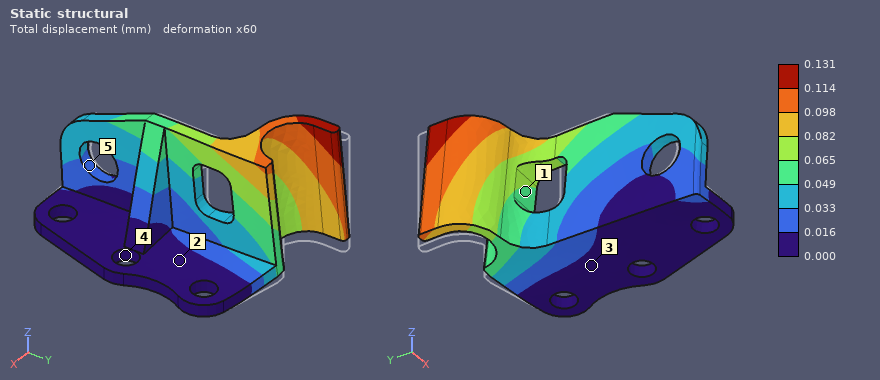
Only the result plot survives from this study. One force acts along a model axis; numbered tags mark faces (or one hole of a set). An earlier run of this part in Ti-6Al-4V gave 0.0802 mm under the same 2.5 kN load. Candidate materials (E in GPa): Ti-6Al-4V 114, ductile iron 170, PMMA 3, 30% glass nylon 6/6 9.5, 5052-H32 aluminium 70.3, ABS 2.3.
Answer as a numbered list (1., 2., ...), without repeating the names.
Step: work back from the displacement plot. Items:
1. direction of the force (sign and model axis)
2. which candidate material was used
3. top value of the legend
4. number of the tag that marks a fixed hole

1. -Y
2. 5052-H32 aluminium
3. 0.131 mm
4. 4
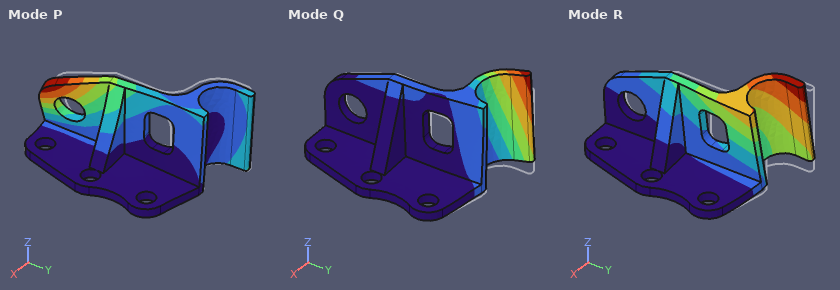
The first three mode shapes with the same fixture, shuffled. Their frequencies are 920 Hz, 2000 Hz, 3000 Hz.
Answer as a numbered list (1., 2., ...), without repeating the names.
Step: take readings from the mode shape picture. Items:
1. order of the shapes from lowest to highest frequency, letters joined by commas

1. R, Q, P
